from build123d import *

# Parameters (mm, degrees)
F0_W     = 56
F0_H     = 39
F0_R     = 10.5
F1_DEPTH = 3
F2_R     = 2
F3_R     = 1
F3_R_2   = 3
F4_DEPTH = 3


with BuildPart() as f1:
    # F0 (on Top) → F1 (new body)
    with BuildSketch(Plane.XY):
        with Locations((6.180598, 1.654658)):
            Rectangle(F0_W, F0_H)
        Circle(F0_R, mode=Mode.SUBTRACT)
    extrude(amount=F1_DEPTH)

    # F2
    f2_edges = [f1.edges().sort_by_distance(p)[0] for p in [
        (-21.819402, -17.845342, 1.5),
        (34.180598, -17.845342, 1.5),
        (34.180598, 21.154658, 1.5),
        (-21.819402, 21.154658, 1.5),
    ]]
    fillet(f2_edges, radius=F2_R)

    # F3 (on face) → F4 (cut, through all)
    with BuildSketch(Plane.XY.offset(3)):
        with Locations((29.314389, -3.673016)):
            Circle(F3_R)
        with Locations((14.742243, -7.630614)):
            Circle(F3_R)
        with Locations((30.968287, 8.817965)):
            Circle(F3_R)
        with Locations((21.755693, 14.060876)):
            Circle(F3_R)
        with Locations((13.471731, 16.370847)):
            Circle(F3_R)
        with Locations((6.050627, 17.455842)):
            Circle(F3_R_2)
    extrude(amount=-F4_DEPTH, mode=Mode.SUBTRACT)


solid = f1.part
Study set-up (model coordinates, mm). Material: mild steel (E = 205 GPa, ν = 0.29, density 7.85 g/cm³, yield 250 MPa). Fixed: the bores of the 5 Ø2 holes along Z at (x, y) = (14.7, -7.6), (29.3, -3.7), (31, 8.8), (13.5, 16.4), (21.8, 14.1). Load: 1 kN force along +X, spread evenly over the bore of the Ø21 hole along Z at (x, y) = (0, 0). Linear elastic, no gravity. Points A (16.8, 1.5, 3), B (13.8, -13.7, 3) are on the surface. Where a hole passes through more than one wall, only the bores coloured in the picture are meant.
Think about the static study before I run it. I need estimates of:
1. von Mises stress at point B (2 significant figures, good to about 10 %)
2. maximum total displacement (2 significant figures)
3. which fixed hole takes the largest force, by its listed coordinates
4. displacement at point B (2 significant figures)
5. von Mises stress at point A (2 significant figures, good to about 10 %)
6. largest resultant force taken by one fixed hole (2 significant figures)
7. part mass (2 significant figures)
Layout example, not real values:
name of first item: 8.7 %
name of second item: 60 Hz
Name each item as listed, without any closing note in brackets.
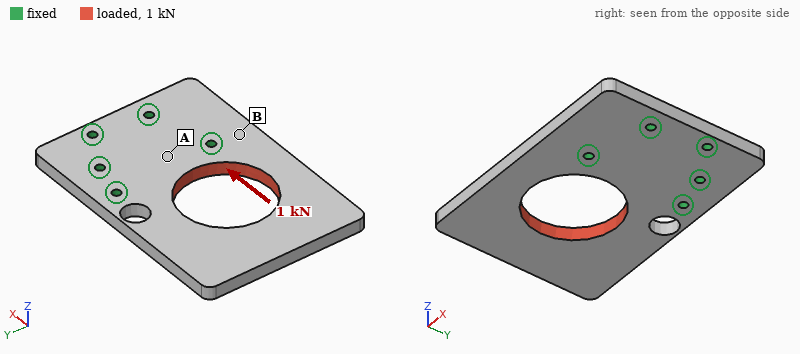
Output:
von Mises stress at point B: 11 MPa
maximum total displacement: 3.2 µm
which fixed hole takes the largest force, by its listed coordinates: (14.7, -7.6)
displacement at point B: 0.85 µm
von Mises stress at point A: 4.5 MPa
largest resultant force taken by one fixed hole: 470 N
part mass: 42 g
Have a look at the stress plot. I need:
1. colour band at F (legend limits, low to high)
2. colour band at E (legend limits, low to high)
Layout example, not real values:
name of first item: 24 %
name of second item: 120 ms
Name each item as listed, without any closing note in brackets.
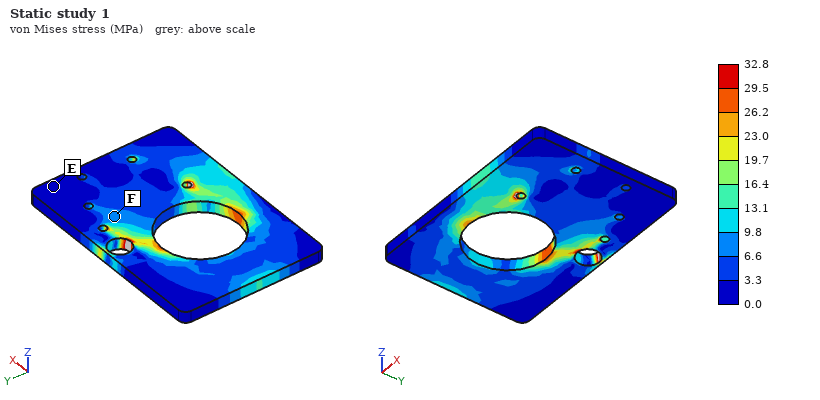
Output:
colour band at F: 6.6 to 9.8 MPa
colour band at E: 0.0 to 3.3 MPa
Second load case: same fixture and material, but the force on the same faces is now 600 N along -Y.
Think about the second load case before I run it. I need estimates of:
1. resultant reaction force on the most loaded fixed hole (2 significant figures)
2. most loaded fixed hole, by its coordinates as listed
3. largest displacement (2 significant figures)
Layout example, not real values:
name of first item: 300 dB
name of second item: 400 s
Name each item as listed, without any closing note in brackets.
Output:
resultant reaction force on the most loaded fixed hole: 450 N
most loaded fixed hole, by its coordinates as listed: (14.7, -7.6)
largest displacement: 8.9 µm
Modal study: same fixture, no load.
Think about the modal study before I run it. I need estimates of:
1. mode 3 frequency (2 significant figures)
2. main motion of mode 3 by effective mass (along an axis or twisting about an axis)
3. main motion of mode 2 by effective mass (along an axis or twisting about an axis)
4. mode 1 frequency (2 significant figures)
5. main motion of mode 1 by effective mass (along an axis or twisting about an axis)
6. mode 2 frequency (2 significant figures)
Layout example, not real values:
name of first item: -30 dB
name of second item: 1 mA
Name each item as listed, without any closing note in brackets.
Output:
mode 3 frequency: 8000 Hz
main motion of mode 3 by effective mass: along Y
main motion of mode 2 by effective mass: twisting about X
mode 1 frequency: 1400 Hz
main motion of mode 1 by effective mass: along Z
mode 2 frequency: 3400 Hz
